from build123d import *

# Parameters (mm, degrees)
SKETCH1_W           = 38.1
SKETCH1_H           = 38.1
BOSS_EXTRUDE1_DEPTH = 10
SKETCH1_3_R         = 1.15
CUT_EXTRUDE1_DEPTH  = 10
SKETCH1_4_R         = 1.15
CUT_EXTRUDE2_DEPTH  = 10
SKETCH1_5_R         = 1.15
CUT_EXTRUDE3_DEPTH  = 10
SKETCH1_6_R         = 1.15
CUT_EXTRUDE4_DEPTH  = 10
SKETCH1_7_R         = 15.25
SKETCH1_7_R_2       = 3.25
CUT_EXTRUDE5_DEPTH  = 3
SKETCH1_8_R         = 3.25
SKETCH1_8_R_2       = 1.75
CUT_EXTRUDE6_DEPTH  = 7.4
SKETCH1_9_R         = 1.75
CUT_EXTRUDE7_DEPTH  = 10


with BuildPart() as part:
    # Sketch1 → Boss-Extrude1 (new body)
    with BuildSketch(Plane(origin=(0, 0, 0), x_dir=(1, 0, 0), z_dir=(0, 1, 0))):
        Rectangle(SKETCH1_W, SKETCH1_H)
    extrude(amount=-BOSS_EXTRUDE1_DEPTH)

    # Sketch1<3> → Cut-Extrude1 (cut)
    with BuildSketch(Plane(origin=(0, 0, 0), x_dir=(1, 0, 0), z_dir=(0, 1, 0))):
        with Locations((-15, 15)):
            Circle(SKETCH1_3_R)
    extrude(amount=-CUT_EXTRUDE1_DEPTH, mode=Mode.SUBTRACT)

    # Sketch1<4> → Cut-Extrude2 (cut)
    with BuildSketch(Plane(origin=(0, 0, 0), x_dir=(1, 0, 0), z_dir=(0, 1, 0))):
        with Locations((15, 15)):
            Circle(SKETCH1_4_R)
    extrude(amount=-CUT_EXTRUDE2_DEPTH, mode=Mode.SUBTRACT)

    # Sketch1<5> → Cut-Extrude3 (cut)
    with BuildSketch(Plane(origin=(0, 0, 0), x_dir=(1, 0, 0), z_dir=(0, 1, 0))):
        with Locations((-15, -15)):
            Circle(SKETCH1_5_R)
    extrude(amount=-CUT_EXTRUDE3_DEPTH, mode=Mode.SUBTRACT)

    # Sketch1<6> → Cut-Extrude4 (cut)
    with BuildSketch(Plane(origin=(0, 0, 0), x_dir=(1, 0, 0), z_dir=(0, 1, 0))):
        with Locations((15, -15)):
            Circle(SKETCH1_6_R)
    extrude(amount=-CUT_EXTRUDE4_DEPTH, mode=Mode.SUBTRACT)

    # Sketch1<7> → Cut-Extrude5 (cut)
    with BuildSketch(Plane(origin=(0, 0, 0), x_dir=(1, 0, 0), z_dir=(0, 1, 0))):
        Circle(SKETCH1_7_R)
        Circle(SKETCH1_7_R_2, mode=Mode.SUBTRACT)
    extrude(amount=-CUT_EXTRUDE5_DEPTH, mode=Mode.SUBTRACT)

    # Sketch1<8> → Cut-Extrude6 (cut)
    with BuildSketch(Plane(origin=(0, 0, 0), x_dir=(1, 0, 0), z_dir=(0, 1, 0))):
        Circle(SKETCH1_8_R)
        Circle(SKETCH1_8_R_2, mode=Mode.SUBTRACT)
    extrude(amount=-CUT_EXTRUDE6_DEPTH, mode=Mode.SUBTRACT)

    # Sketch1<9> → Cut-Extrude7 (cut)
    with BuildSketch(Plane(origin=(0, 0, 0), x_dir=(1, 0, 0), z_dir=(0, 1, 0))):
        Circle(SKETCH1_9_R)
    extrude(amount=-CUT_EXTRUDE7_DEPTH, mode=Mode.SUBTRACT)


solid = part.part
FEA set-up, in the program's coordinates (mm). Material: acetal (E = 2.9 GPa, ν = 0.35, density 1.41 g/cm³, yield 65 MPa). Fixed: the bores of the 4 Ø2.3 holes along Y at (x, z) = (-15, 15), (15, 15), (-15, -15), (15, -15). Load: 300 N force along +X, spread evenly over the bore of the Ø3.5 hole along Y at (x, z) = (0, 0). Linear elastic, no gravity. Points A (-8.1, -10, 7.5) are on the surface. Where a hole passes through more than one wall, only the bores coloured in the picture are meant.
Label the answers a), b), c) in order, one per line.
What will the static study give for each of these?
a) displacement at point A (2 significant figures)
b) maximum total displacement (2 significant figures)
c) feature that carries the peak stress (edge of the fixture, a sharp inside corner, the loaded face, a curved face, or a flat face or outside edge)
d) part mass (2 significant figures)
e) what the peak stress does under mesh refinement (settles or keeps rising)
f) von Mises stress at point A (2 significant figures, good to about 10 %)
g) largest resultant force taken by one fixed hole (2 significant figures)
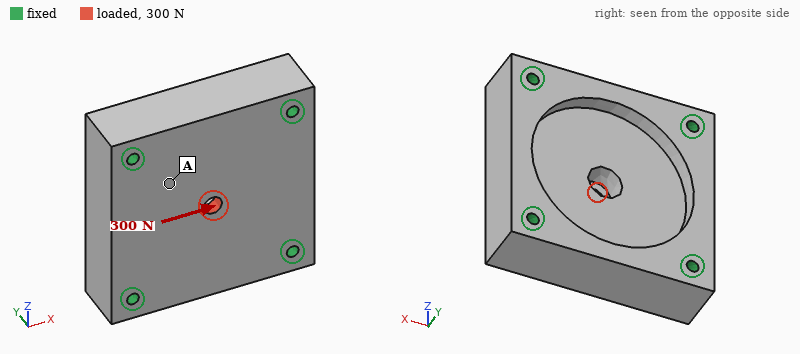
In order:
a) 5.8 µm
b) 24 µm
c) a sharp inside corner
d) 17 g
e) keeps rising
f) 1.7 MPa
g) 86 N
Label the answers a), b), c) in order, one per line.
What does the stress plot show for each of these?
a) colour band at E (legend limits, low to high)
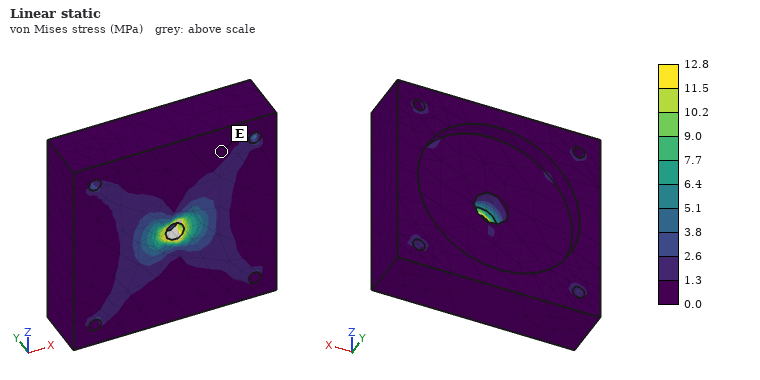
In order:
a) 0.0 to 1.3 MPa
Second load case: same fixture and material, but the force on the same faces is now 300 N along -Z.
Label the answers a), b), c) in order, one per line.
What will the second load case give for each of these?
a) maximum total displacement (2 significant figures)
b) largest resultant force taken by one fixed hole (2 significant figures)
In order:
a) 23 µm
b) 86 N
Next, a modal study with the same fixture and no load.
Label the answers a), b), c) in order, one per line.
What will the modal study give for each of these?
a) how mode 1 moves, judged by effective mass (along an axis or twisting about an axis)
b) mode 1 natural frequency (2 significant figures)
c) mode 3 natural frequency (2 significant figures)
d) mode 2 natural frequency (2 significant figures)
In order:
a) along Y
b) 7200 Hz
c) 10 kHz
d) 10 kHz
